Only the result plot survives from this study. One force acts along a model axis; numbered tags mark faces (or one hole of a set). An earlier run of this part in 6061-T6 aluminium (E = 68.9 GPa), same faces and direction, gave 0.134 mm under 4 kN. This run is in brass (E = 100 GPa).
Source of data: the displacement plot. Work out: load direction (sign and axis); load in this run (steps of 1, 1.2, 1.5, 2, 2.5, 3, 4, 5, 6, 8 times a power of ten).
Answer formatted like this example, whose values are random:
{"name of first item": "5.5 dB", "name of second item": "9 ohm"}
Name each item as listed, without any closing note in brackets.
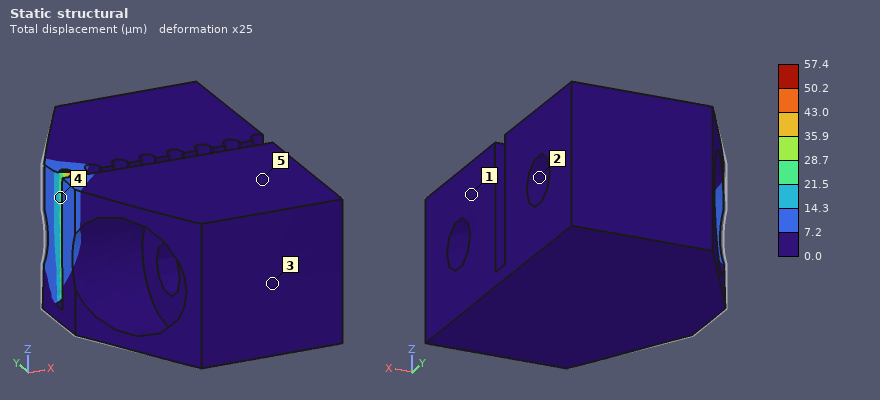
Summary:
{"load direction": "+X", "load in this run": "2.5 kN"}
